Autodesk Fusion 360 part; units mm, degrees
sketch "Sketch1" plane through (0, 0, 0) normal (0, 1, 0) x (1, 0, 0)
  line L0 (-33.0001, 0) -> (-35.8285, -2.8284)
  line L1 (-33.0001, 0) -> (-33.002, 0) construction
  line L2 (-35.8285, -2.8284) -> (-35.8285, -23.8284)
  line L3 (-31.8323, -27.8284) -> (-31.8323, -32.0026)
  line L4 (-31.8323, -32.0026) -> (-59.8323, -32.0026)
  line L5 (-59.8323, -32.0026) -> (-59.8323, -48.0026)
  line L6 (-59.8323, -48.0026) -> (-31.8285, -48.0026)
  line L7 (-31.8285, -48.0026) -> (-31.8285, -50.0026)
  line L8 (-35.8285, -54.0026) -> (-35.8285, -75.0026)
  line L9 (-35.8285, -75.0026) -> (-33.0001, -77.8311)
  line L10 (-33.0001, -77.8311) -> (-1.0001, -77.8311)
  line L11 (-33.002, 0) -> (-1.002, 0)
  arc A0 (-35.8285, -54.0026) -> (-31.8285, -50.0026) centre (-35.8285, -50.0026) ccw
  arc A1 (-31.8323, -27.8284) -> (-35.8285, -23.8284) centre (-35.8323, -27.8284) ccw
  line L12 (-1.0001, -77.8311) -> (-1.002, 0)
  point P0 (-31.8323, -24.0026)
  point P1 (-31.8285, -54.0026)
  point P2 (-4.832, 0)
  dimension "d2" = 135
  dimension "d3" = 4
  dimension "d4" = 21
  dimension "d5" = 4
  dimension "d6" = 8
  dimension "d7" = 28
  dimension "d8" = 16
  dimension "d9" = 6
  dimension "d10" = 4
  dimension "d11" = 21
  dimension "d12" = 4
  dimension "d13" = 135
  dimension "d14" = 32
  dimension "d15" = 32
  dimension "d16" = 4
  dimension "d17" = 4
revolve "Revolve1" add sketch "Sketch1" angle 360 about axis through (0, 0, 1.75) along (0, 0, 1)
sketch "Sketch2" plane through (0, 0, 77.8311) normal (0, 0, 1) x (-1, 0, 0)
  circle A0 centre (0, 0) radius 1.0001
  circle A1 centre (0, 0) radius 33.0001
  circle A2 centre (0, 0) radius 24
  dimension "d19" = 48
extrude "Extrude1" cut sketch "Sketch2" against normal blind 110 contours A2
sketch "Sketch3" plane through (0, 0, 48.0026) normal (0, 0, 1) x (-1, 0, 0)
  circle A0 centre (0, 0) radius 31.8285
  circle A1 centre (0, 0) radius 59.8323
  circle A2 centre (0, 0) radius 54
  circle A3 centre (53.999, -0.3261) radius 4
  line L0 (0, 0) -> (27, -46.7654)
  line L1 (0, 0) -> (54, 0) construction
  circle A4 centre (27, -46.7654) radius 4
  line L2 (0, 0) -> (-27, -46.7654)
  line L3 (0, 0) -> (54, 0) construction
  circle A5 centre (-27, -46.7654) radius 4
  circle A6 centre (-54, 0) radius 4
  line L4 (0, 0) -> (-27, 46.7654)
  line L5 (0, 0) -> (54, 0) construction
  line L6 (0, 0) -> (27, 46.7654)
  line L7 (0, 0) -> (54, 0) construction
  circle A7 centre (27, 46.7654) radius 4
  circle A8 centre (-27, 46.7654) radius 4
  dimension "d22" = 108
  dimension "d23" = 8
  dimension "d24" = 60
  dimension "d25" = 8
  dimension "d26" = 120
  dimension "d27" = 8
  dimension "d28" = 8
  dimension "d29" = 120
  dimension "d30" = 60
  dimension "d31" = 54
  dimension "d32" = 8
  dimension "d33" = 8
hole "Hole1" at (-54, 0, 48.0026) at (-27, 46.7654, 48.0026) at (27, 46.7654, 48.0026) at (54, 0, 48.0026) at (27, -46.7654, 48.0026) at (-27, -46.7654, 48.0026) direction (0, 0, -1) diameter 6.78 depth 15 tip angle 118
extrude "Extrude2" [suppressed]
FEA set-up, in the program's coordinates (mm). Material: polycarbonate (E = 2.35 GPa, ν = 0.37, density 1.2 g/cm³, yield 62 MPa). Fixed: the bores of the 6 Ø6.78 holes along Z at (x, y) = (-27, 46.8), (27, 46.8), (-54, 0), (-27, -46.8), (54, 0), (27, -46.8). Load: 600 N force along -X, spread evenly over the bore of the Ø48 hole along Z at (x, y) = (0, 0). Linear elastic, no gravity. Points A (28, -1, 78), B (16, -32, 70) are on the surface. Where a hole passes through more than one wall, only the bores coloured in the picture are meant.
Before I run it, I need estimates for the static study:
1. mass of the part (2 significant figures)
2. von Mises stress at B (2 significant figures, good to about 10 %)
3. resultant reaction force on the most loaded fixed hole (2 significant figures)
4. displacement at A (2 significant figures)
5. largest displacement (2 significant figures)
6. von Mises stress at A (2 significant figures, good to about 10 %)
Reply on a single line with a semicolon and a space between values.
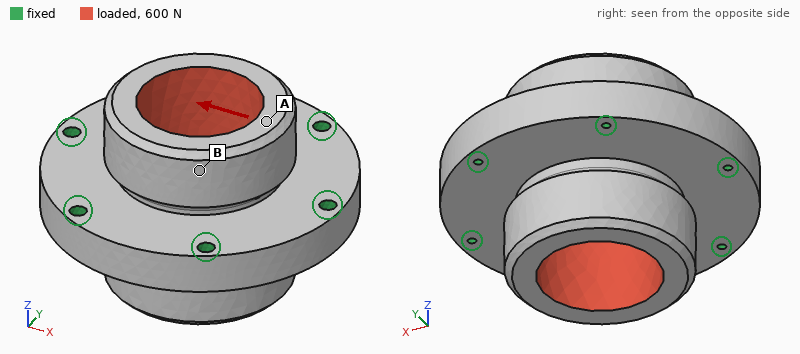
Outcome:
330 g; 0.065 MPa; 130 N; 12 µm; 14 µm; 0.22 MPa
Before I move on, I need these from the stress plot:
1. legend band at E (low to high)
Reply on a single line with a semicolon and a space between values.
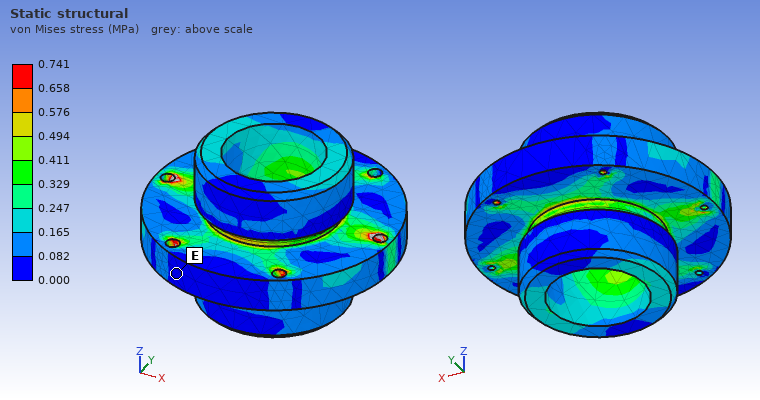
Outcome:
0.000 to 0.082 MPa
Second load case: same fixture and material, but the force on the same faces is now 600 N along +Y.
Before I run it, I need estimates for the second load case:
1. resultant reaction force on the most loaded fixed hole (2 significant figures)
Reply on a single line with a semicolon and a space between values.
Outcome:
120 N
